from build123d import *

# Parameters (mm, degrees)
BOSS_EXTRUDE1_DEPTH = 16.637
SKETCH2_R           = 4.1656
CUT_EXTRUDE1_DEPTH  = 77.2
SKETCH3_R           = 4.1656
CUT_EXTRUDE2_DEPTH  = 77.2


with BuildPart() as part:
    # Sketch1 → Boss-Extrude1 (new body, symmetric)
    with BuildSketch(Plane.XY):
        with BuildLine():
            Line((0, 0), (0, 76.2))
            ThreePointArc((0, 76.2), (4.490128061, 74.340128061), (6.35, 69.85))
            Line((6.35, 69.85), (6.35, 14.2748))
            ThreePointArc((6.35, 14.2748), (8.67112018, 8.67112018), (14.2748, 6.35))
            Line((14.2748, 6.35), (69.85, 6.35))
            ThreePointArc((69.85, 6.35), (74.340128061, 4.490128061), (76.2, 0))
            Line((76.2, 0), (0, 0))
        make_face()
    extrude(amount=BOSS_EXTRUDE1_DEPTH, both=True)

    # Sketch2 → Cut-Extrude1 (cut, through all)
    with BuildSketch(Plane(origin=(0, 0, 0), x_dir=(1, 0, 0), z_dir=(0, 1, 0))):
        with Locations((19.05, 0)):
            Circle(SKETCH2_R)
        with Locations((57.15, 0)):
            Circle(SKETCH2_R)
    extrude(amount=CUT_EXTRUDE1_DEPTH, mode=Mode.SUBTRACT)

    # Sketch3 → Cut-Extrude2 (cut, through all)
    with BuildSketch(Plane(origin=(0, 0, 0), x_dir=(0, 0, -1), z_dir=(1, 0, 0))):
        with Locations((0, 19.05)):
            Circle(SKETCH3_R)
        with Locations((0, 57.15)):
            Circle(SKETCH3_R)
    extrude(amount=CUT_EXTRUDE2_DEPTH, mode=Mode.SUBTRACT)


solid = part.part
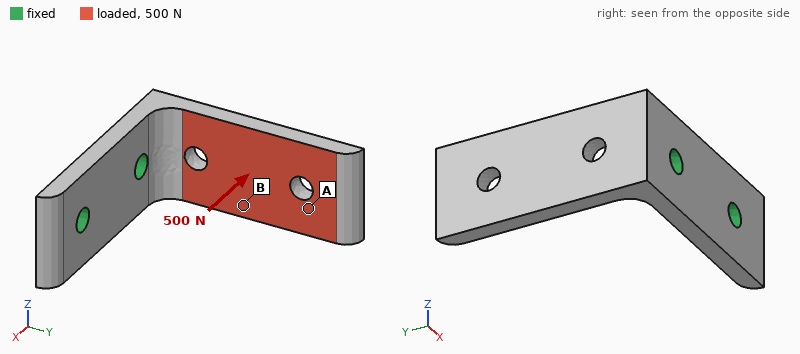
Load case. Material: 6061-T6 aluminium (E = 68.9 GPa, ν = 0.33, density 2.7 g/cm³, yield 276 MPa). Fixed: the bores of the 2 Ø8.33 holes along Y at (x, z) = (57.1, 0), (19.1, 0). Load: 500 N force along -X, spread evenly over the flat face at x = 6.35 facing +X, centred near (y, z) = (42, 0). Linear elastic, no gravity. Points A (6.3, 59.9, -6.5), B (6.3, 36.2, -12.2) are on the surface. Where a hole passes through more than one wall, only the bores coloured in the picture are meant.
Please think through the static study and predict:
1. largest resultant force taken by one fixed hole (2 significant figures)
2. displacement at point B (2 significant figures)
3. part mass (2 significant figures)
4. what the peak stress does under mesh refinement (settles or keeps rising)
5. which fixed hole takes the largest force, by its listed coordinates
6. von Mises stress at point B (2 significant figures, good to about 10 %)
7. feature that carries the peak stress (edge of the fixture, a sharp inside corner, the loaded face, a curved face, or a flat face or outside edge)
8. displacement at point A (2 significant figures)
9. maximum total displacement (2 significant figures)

480 N
0.23 mm
79 g
keeps rising
(19.1, 0)
24 MPa
edge of the fixture
0.50 mm
0.70 mm
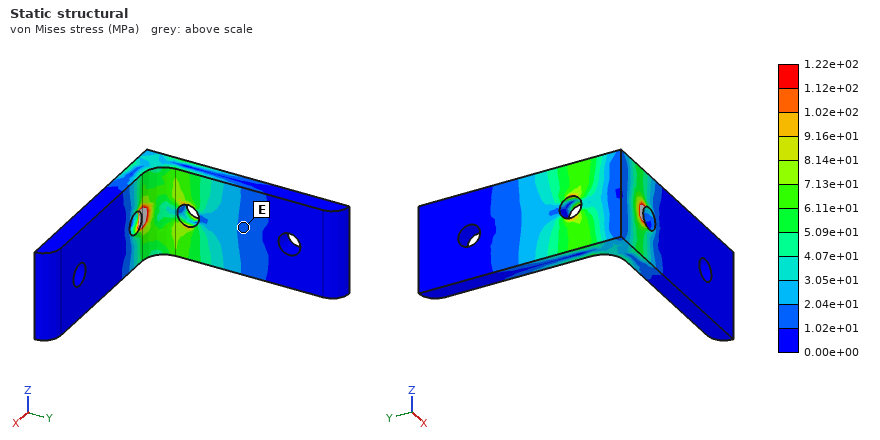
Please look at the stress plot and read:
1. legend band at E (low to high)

1.02e+01 to 2.04e+01 MPa
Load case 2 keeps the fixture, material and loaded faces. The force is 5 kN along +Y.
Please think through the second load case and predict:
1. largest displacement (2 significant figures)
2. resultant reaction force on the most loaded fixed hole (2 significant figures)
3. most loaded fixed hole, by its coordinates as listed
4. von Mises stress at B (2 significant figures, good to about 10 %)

0.14 mm
5.2 kN
(19.1, 0)
61 MPa
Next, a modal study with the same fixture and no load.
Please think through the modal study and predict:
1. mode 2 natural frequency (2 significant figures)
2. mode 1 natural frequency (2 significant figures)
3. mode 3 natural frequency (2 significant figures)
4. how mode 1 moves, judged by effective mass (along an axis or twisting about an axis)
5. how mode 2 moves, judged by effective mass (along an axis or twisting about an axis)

1700 Hz
880 Hz
4200 Hz
along X
along Z
